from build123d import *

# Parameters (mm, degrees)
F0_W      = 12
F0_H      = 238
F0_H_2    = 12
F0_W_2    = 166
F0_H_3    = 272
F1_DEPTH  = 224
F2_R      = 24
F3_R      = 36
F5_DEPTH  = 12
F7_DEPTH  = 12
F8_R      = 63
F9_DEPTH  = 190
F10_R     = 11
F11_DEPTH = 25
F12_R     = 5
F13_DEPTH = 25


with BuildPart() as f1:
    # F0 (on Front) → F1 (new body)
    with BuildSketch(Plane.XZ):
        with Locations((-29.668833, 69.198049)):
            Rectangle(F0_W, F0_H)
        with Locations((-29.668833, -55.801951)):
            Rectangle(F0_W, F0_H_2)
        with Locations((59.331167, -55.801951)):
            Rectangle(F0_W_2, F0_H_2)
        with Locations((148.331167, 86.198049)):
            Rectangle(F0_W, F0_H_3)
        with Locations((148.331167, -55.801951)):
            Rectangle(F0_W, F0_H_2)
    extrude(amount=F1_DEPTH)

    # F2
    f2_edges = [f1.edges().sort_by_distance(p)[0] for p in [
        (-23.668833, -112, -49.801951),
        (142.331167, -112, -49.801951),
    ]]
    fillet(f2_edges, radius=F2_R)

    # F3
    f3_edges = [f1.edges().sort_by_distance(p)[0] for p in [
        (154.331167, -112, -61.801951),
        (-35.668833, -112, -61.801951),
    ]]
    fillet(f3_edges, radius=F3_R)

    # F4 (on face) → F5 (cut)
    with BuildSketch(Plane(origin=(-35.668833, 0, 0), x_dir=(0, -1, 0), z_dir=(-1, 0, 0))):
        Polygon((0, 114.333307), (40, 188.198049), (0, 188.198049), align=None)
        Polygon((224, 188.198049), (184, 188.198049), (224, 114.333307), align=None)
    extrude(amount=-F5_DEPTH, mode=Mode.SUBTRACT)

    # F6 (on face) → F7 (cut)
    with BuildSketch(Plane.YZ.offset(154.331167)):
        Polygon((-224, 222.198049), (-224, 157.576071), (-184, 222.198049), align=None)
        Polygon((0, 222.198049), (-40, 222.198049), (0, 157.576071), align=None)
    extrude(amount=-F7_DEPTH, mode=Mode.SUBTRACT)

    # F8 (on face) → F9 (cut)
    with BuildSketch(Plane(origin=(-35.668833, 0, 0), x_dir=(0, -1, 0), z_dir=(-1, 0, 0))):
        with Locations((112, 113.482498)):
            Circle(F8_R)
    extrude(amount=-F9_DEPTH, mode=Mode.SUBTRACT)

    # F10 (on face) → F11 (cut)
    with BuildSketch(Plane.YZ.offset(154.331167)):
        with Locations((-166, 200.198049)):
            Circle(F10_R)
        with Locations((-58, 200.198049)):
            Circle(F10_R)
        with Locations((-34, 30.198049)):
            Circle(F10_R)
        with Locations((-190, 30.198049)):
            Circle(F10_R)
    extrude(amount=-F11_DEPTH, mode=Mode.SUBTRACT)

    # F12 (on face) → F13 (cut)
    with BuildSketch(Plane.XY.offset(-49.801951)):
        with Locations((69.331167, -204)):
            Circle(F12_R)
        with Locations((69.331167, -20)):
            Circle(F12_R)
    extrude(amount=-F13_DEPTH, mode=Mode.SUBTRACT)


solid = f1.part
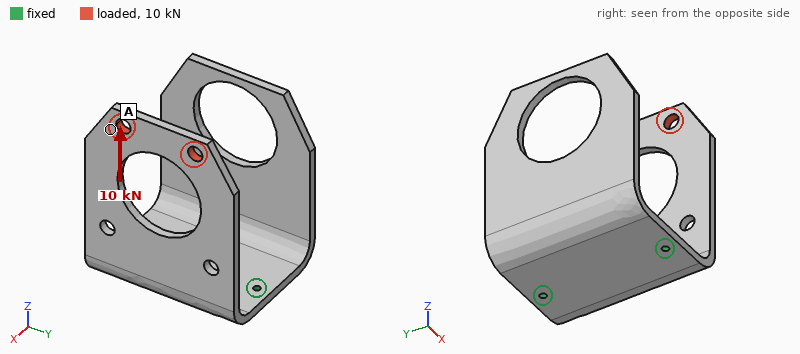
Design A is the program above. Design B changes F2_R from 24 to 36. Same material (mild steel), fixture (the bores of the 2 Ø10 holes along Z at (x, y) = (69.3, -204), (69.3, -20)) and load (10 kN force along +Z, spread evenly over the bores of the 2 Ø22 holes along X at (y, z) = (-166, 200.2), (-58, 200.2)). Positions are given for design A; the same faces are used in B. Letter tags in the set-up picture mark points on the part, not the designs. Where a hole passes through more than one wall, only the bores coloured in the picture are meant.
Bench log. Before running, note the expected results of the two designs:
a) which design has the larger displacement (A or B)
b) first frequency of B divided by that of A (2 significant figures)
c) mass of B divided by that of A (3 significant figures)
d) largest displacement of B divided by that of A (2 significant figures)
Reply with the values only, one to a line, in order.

A
1.1
1.05
0.92
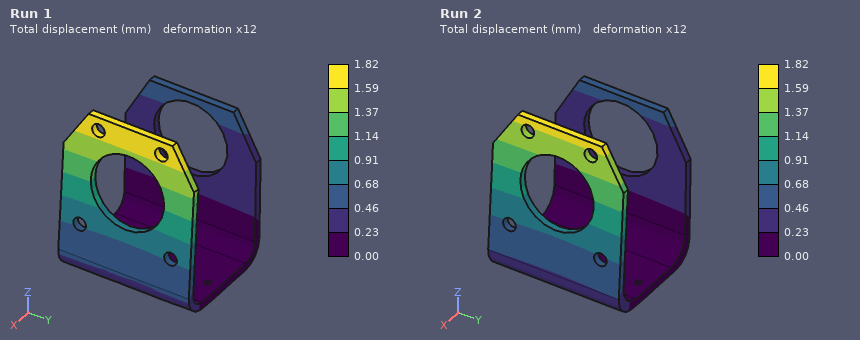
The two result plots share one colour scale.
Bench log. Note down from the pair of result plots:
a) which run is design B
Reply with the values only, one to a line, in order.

Run 2
